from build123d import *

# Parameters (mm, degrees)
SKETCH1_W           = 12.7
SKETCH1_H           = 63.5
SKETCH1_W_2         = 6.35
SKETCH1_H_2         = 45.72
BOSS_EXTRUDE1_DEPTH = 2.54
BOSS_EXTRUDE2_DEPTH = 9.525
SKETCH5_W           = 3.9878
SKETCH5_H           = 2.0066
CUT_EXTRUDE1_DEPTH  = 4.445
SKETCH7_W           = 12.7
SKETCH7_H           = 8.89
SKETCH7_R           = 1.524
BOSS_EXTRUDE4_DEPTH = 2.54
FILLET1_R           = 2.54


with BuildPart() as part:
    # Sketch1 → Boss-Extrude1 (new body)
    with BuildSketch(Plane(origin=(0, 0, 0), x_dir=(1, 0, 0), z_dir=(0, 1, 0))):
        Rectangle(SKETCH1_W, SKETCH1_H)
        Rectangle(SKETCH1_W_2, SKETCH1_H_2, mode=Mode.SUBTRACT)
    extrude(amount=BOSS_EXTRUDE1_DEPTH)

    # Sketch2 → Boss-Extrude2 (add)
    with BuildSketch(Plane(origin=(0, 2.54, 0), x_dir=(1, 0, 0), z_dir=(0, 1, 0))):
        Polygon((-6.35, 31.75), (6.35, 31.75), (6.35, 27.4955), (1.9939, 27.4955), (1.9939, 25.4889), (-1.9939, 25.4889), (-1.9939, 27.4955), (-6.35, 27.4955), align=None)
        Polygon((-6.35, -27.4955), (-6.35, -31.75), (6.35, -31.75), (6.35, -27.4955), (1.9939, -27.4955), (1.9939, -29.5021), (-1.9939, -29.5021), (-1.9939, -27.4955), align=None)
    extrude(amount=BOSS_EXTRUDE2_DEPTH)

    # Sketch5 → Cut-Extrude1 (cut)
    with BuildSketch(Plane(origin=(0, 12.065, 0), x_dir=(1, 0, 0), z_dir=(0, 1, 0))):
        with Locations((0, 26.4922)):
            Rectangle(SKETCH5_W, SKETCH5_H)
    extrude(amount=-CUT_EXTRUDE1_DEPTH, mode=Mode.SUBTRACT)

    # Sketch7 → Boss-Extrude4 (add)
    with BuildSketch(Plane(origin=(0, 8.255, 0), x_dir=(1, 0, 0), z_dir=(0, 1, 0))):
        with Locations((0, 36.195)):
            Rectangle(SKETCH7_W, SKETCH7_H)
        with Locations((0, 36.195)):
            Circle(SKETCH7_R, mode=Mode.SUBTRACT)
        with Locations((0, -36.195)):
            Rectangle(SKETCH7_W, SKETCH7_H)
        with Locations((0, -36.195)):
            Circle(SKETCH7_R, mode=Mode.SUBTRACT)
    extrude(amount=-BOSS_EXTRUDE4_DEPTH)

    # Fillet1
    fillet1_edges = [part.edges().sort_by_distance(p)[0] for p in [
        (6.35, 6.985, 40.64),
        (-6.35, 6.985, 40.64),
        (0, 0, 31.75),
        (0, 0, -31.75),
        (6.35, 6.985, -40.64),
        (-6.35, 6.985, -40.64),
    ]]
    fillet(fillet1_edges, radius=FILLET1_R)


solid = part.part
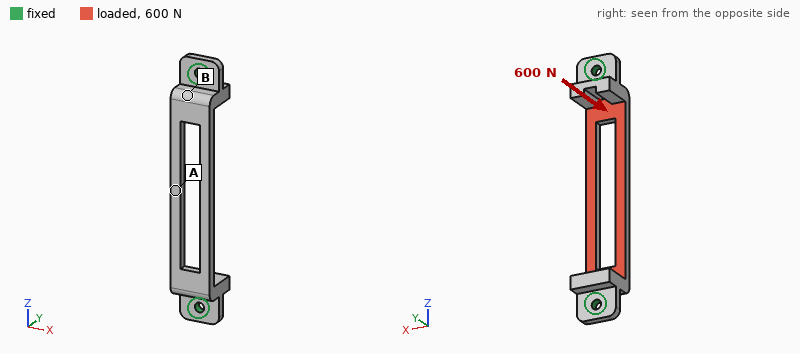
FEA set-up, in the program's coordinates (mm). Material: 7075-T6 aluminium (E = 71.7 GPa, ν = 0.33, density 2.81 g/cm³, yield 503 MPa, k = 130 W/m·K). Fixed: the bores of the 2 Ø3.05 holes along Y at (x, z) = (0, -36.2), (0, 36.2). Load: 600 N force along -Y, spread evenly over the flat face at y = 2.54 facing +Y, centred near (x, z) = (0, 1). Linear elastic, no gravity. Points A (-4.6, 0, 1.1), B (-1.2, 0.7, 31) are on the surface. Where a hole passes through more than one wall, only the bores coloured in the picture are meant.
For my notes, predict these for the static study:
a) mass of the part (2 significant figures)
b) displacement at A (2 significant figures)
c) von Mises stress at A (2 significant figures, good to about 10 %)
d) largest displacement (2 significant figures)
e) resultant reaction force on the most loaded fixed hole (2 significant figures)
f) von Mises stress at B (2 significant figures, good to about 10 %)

7.8 g
0.40 mm
210 MPa
0.40 mm
690 N
33 MPa
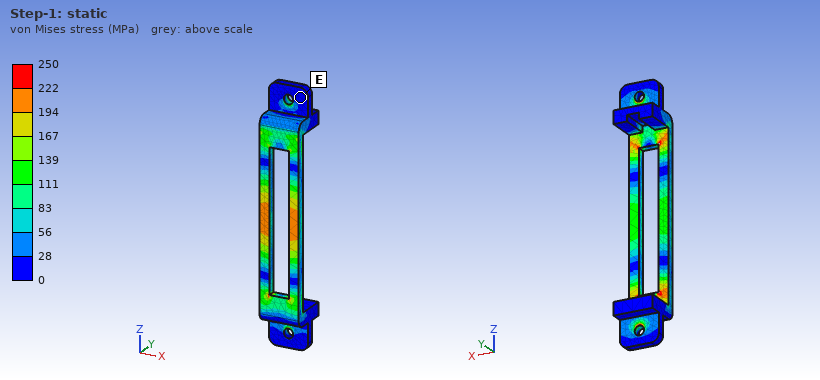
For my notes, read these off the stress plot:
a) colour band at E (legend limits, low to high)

0 to 28 MPa
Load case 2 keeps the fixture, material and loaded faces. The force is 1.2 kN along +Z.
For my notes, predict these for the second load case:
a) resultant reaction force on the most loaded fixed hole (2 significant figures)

600 N
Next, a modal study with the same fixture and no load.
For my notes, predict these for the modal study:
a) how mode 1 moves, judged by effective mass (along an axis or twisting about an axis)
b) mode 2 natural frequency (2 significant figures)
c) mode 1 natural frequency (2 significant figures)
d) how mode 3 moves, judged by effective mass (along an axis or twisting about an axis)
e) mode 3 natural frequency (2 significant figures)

along Y
4600 Hz
4200 Hz
along X
5700 Hz
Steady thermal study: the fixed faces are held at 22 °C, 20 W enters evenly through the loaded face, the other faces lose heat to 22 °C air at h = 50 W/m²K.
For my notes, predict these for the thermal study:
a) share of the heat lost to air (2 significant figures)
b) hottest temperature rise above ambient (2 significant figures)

15 %
63 K
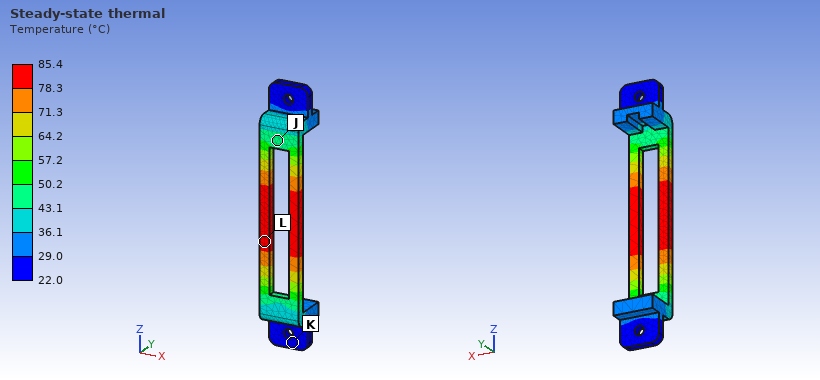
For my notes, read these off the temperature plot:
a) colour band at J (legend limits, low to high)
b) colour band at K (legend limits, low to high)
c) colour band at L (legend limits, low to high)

43.1 to 50.2 °C
22.0 to 29.0 °C
78.3 to 85.4 °C
